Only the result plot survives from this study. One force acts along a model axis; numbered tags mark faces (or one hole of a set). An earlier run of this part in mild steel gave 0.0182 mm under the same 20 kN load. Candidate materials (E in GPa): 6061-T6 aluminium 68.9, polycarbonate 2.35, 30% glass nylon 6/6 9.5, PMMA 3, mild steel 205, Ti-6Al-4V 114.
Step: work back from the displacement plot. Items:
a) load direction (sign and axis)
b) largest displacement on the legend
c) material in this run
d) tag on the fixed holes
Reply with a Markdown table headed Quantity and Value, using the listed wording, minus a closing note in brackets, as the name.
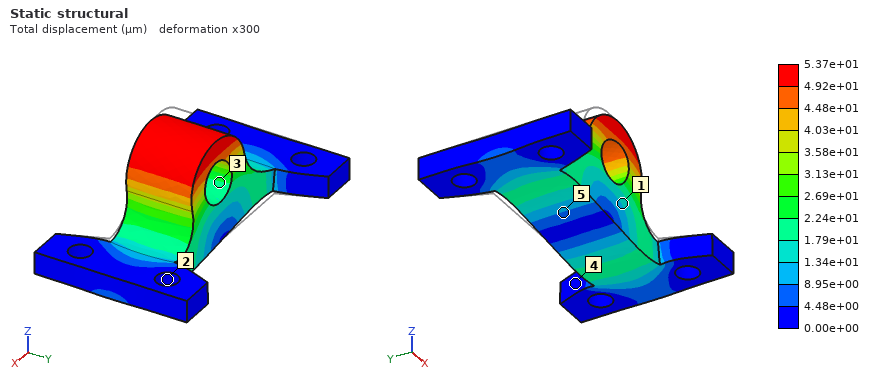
| Quantity | Value |
|---|---|
| load direction | +X |
| largest displacement on the legend | 5.37e+01 µm |
| material in this run | 6061-T6 aluminium |
| tag on the fixed holes | 2 |
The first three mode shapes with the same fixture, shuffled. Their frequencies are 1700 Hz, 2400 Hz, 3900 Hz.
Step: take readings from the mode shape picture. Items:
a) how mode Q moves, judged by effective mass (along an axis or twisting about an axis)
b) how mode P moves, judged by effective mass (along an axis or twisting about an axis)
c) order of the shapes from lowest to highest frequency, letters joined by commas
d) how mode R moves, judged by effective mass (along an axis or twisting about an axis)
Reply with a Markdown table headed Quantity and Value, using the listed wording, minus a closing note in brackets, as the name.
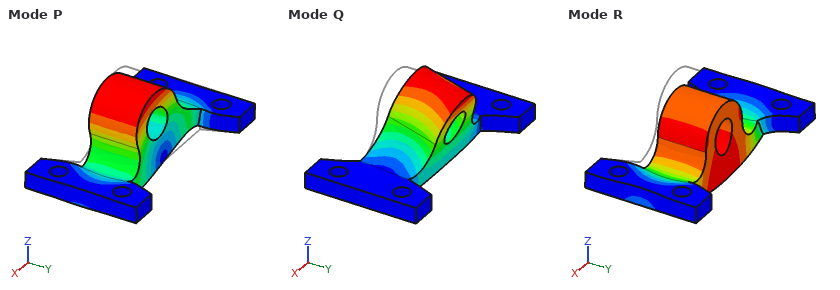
| Quantity | Value |
|---|---|
| how mode Q moves, judged by effective mass | along Y |
| how mode P moves, judged by effective mass | along X |
| order of the shapes from lowest to highest frequency, letters joined by commas | Q, R, P |
| how mode R moves, judged by effective mass | along Z |
